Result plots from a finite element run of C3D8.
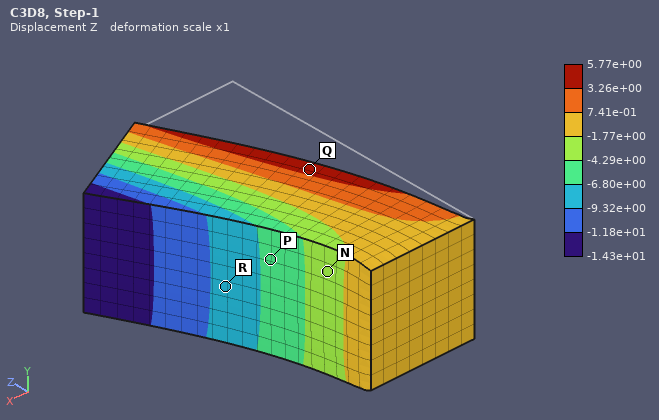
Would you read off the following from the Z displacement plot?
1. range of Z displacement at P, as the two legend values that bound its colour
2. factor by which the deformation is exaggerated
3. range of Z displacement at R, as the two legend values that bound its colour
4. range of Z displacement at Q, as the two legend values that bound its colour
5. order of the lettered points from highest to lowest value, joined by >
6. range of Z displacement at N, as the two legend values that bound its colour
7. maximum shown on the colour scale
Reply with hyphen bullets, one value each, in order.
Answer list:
- -6.80e+00 to -4.29e+00
- 1
- -9.32e+00 to -6.80e+00
- 3.26e+00 to 5.77e+00
- Q > N > P > R
- -4.29e+00 to -1.77e+00
- 5.77e+00
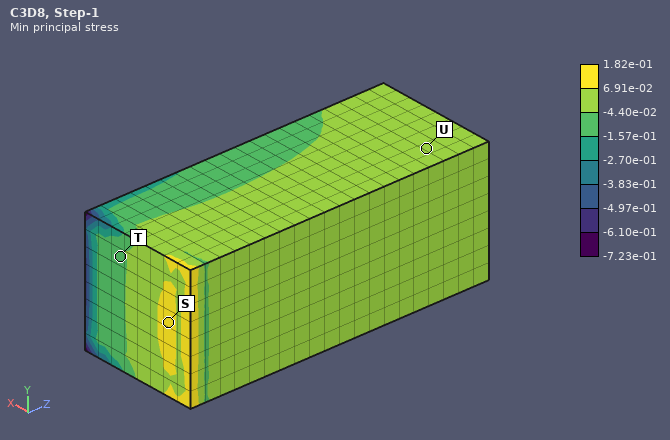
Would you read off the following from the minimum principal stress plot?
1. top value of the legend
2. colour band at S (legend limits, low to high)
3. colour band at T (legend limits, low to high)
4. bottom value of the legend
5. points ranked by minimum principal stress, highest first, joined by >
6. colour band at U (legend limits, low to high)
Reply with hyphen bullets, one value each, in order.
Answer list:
- 1.82e-01
- 6.91e-02 to 1.82e-01
- -1.57e-01 to -4.40e-02
- -7.23e-01
- S > U > T
- -4.40e-02 to 6.91e-02
